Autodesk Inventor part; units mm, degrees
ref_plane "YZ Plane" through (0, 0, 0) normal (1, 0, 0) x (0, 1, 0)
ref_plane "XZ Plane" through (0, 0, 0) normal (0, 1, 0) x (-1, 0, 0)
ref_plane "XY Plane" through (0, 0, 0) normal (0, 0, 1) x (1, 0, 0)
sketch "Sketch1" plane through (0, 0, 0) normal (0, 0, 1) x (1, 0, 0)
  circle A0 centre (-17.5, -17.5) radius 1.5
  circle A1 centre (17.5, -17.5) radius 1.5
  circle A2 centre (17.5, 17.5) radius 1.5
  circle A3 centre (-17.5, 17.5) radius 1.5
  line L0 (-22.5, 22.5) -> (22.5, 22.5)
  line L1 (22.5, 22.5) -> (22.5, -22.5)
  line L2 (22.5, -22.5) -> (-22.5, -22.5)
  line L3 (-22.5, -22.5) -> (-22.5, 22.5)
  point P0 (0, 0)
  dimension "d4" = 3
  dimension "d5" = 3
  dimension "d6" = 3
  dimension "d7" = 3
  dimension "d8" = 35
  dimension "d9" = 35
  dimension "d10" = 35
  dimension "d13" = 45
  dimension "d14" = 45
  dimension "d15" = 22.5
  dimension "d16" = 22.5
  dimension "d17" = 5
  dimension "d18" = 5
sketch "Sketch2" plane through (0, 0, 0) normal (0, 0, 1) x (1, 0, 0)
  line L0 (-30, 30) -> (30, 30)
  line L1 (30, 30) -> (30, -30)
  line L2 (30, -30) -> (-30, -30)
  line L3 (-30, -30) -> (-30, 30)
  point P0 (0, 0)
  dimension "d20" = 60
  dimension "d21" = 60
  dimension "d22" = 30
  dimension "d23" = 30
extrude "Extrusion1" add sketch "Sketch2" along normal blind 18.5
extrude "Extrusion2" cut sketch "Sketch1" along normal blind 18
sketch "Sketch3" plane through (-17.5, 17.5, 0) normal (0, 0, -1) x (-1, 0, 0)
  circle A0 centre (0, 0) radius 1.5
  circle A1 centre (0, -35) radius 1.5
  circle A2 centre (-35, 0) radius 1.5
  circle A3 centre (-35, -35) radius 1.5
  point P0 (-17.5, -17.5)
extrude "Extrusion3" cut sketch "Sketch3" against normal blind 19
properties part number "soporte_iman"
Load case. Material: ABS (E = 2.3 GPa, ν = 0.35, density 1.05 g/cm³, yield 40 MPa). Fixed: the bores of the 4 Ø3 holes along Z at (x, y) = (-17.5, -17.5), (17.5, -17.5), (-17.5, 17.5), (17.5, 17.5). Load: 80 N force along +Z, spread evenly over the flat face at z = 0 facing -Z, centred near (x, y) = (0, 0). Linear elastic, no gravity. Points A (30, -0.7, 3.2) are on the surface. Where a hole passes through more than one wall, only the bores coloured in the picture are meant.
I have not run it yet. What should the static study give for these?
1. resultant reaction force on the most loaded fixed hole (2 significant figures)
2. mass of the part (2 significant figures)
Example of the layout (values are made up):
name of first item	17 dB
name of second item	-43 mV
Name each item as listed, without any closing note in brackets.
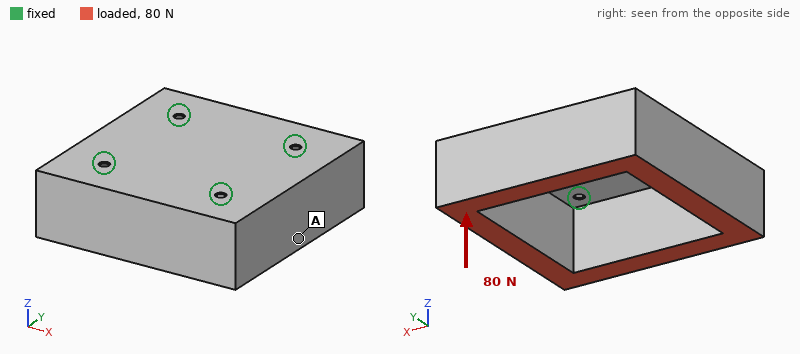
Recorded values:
resultant reaction force on the most loaded fixed hole	21 N
mass of the part	32 g
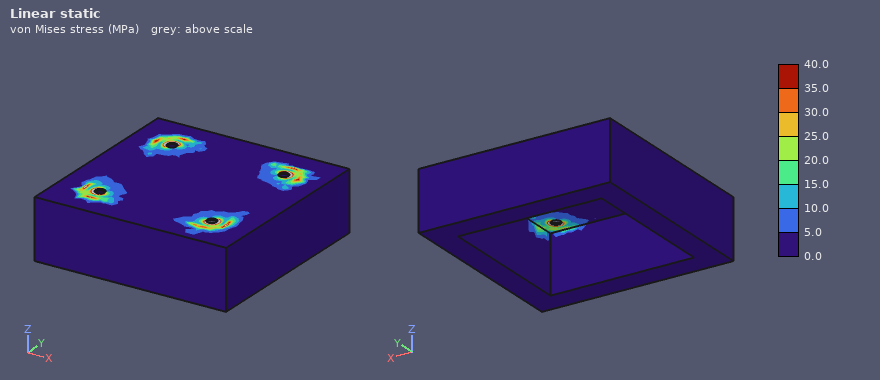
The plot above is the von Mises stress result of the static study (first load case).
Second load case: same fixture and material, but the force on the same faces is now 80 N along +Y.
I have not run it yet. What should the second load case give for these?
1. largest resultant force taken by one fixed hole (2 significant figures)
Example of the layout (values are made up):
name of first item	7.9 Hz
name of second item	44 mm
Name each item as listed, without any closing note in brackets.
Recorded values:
largest resultant force taken by one fixed hole	29 N
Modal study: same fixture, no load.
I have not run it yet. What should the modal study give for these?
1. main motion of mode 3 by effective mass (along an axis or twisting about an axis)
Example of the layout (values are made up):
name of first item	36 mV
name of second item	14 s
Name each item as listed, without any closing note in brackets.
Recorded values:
main motion of mode 3 by effective mass	along Z
